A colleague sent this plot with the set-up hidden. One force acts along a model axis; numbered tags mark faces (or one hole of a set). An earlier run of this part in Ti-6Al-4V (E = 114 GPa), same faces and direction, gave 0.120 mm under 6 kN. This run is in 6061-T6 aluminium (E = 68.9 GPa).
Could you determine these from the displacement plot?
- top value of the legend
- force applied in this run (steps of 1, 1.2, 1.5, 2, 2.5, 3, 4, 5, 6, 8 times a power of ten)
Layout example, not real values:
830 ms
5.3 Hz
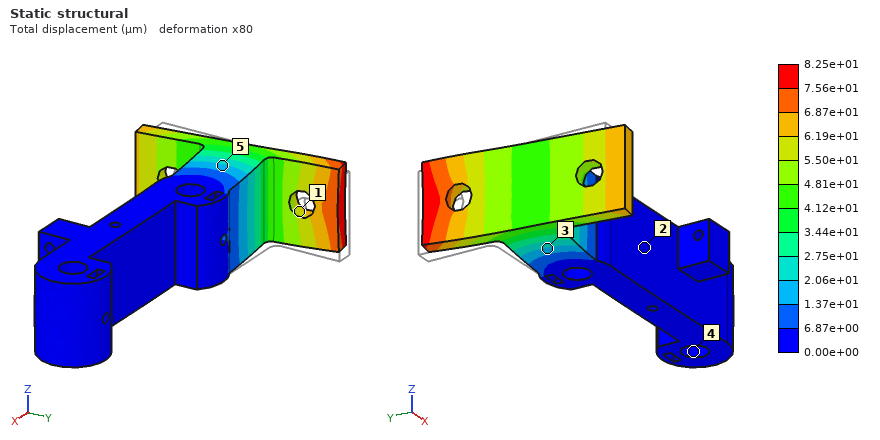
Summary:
8.25e+01 µm
2.5 kN
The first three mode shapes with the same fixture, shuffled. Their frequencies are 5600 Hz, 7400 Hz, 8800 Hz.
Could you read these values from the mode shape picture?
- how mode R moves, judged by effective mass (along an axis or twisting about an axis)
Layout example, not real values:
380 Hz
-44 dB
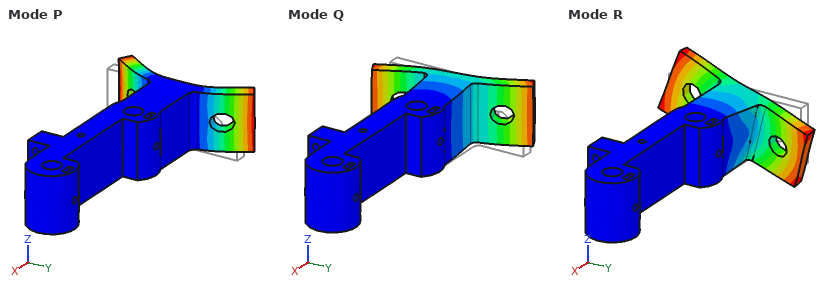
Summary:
twisting about X
